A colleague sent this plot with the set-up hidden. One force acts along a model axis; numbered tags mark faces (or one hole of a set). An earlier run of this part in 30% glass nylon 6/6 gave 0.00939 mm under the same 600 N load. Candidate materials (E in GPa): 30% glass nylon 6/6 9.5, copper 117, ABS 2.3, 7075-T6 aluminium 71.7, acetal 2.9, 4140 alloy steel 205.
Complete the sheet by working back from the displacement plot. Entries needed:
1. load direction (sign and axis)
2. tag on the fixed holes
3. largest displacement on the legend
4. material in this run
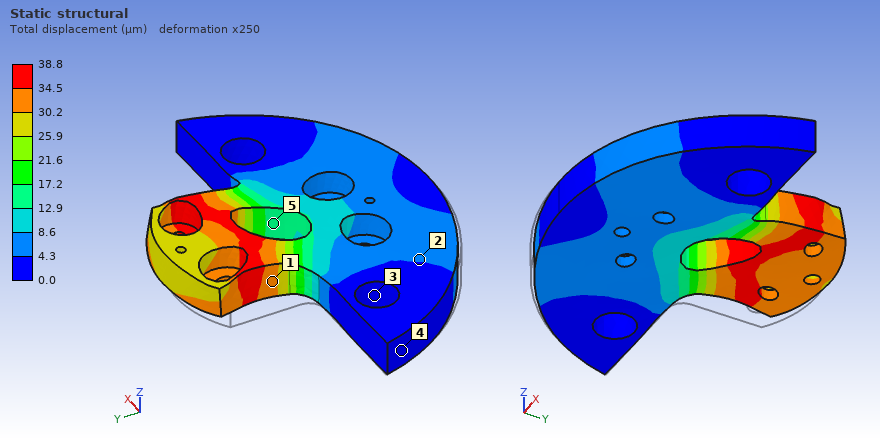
+X
3
38.8 µm
ABS
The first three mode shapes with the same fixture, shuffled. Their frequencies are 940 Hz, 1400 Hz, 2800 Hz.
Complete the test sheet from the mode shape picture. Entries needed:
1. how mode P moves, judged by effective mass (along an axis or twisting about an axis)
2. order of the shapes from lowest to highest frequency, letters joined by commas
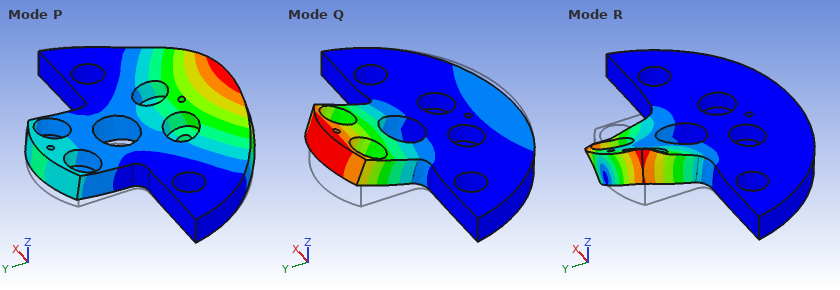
along Z
Q, P, R
